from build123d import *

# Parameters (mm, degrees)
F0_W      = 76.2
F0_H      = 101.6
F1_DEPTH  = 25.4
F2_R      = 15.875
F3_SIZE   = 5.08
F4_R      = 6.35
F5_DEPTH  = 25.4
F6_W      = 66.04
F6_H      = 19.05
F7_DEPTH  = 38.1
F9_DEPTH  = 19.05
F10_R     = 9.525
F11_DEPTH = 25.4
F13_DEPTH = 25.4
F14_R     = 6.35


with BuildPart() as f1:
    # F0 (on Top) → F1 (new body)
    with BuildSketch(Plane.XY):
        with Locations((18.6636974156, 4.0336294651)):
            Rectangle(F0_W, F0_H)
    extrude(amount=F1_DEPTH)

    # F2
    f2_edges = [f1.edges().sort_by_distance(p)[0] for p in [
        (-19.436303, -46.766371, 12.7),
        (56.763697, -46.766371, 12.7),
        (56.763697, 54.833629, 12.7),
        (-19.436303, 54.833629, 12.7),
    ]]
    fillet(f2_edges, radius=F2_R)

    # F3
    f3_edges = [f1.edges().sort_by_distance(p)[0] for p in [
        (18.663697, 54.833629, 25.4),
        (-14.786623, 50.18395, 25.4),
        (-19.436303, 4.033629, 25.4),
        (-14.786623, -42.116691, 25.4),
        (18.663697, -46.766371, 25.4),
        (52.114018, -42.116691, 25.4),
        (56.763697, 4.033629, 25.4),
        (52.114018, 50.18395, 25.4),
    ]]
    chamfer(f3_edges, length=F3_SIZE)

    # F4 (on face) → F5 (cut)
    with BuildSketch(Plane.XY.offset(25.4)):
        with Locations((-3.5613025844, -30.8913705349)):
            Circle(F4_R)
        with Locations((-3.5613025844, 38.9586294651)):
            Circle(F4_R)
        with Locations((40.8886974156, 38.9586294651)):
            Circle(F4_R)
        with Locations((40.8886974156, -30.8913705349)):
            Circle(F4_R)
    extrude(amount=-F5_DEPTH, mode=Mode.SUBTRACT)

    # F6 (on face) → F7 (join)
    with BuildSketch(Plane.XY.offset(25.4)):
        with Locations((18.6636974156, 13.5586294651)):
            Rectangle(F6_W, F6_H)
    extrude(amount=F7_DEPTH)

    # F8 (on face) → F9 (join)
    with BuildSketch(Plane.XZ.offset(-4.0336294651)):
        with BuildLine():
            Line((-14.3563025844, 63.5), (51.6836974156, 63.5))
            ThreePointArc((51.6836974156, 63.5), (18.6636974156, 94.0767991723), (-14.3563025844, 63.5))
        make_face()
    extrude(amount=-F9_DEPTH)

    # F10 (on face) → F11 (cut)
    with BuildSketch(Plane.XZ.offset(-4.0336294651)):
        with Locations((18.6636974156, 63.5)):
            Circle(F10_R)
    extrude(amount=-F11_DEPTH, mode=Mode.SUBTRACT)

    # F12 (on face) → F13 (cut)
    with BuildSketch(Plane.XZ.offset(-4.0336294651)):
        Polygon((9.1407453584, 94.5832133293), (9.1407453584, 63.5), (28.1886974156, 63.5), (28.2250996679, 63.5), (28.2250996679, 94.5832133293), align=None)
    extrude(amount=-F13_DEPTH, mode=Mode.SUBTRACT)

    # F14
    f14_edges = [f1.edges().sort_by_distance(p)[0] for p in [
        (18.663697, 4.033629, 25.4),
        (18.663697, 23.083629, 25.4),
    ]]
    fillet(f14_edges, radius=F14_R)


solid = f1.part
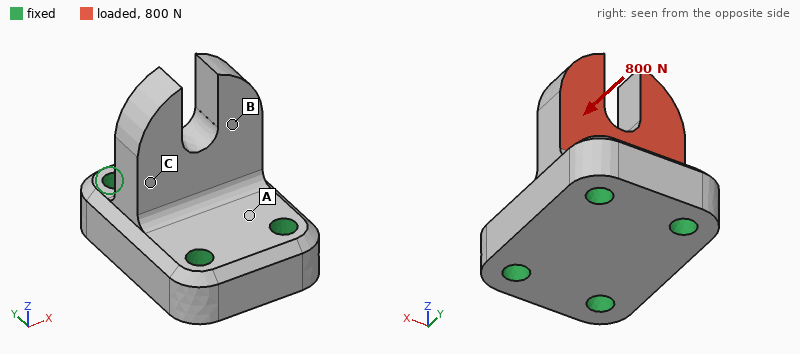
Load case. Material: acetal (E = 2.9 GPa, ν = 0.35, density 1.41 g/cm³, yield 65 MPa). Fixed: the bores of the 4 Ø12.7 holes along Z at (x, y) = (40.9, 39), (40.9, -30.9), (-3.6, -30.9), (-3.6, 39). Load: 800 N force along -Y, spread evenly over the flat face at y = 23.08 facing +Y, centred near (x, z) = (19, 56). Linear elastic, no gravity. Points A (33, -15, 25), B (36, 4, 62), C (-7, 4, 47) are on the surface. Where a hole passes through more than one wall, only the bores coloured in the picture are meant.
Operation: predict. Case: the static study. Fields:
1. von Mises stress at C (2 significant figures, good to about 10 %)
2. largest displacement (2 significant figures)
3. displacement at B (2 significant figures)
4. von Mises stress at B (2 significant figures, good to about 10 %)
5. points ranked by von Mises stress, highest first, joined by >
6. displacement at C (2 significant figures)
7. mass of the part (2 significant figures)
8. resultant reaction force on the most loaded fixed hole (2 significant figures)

2.6 MPa
0.32 mm
0.15 mm
1.2 MPa
C > B > A
0.083 mm
340 g
390 N
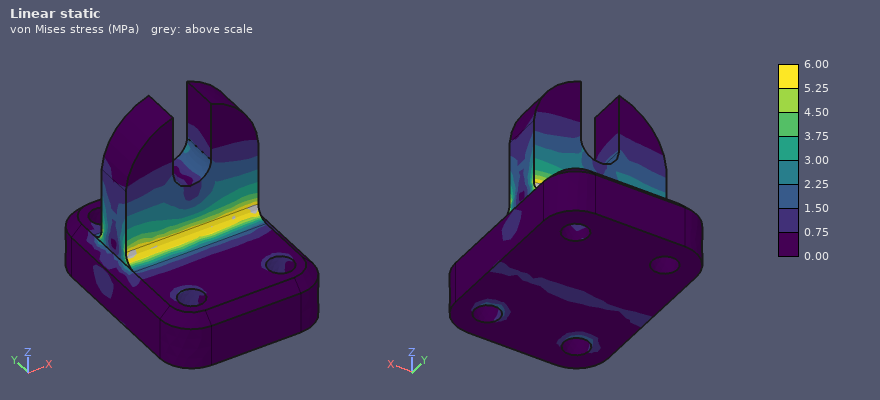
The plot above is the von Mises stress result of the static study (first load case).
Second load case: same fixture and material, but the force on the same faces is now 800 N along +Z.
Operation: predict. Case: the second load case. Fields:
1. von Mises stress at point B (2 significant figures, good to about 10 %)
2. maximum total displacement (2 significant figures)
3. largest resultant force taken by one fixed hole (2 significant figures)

0.63 MPa
0.12 mm
340 N
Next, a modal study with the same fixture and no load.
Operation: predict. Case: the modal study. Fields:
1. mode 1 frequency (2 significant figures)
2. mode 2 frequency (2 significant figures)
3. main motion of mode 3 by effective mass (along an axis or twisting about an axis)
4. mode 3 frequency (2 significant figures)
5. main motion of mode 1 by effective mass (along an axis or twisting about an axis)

1200 Hz
1500 Hz
along X
1800 Hz
along Y
